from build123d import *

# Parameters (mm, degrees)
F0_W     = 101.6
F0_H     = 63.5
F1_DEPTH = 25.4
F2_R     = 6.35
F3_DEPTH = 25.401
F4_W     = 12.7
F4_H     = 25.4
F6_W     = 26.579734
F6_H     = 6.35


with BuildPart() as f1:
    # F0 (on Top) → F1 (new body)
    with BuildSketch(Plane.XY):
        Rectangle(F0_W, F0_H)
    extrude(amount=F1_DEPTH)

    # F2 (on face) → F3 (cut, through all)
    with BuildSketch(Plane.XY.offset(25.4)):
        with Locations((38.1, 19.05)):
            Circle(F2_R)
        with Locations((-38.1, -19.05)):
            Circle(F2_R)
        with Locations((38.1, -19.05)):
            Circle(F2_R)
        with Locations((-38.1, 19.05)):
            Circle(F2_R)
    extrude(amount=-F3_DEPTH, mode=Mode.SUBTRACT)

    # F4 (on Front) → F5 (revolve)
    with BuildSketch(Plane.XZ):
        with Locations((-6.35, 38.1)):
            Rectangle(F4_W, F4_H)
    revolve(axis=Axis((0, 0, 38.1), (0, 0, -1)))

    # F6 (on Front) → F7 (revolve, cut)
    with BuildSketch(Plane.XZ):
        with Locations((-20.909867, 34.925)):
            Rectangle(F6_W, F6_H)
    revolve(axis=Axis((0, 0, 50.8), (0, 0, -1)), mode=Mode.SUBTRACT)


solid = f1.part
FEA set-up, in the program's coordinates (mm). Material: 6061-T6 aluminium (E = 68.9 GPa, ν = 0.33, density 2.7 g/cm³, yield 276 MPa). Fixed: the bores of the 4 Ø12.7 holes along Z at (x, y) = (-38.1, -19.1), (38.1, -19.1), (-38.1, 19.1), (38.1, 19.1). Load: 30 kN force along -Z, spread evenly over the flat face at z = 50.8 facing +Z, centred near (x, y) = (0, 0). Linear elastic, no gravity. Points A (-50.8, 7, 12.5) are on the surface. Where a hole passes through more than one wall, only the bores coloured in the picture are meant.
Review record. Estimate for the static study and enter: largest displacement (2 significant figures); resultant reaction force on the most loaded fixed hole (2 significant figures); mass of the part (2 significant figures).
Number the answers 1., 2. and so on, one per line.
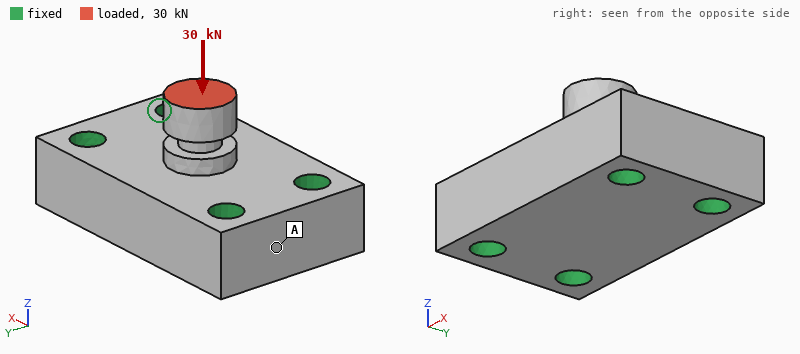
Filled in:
1. 69 µm
2. 7.7 kN
3. 440 g
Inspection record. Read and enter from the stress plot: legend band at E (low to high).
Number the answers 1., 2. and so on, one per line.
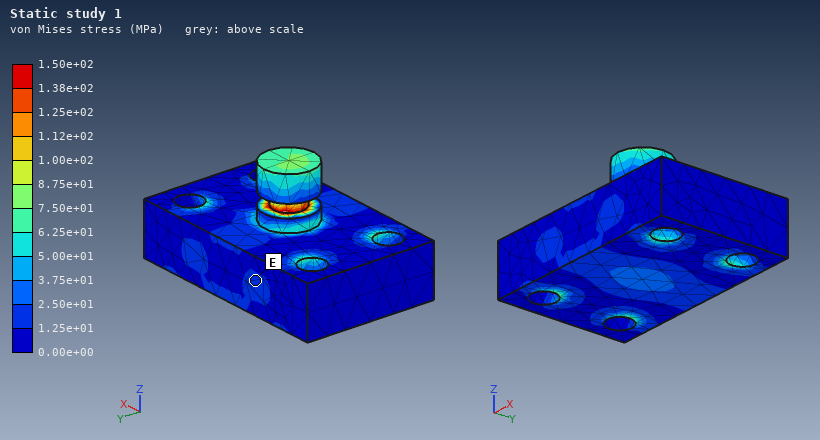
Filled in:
1. 1.25e+01 to 2.50e+01 MPa
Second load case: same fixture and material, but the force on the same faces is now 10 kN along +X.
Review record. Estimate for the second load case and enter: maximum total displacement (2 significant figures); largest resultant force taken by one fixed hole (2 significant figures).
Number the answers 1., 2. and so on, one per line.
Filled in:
1. 0.29 mm
2. 4.2 kN
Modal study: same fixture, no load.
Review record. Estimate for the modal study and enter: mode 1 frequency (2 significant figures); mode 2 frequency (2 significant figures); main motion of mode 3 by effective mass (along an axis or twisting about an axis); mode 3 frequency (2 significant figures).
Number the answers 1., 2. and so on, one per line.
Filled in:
1. 9400 Hz
2. 9900 Hz
3. along Z
4. 15 kHz
